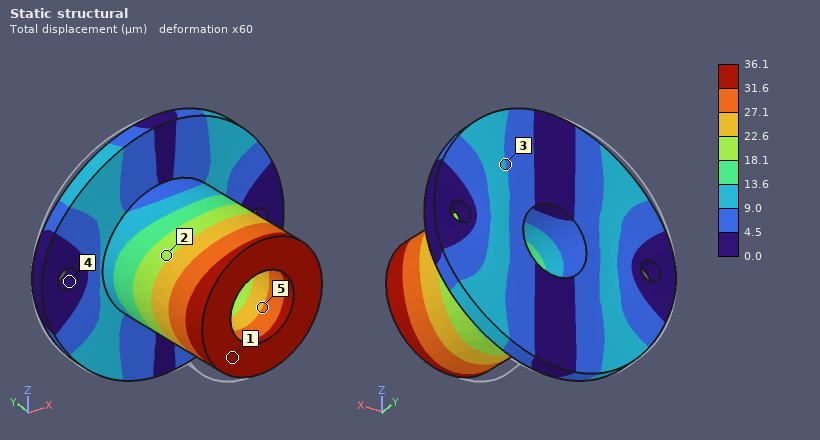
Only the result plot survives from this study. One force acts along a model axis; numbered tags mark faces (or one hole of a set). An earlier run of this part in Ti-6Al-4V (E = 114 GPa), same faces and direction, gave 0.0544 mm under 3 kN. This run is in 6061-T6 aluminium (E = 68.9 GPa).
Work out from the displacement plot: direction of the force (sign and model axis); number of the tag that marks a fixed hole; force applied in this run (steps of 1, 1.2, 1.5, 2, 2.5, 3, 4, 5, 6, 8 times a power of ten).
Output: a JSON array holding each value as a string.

["+X", "4", "1.2 kN"]
